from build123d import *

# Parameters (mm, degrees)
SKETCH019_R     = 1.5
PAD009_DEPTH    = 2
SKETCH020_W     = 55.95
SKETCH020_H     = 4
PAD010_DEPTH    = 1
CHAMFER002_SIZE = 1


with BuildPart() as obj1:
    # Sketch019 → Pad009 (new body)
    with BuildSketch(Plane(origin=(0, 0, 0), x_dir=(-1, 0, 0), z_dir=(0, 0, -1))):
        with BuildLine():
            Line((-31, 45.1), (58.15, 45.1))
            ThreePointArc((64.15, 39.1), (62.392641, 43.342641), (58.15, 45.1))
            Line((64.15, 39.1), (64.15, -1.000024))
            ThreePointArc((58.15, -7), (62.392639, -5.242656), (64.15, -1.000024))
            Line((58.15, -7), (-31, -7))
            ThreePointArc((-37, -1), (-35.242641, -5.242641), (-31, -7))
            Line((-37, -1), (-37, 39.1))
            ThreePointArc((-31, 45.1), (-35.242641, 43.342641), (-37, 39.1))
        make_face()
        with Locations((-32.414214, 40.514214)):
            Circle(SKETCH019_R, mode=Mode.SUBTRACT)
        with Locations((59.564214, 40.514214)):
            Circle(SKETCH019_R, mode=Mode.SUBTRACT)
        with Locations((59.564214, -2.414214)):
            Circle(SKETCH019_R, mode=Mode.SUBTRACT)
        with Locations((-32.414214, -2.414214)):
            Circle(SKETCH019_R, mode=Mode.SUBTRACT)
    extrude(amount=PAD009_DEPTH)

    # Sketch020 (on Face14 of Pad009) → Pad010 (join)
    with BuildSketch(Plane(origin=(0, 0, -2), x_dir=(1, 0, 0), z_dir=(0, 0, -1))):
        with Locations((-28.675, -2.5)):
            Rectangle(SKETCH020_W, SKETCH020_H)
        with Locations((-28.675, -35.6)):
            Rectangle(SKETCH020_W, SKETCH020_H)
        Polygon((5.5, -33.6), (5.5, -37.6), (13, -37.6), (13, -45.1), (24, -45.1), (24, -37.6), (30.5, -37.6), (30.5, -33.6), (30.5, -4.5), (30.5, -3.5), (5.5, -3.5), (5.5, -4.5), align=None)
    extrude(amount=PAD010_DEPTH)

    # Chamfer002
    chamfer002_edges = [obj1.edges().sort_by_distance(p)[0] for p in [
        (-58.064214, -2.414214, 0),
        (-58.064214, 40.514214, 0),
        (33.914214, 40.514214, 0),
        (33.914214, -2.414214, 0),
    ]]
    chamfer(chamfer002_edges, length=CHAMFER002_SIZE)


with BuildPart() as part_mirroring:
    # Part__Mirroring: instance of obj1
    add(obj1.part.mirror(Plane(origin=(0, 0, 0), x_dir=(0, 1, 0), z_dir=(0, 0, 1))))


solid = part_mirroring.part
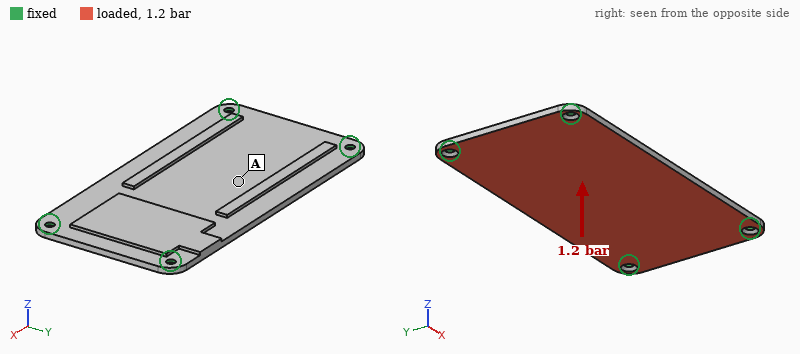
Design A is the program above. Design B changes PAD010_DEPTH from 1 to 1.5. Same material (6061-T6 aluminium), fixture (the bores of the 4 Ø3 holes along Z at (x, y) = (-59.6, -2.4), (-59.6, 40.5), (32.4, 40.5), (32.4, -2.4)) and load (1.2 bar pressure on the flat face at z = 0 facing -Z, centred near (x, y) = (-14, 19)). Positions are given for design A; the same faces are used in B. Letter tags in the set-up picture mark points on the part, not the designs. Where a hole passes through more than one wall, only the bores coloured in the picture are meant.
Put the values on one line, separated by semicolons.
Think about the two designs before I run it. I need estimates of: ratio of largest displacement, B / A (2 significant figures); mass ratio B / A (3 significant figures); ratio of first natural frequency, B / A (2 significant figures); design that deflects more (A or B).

0.88; 1.06; 1.0; A
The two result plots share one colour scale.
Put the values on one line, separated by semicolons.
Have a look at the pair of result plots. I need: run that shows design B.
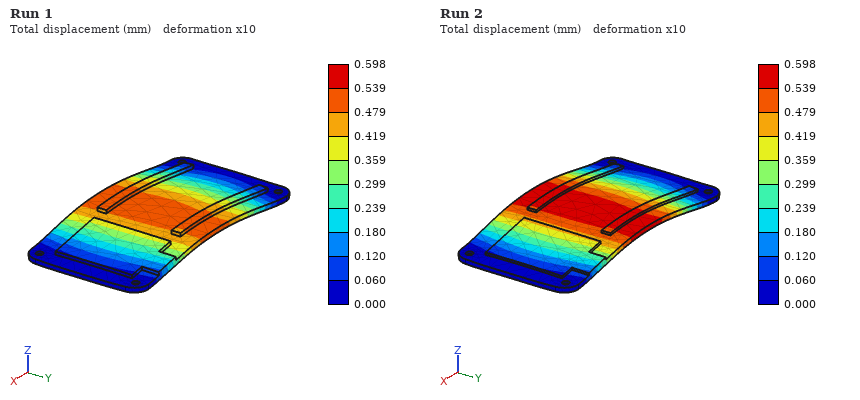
Run 1
